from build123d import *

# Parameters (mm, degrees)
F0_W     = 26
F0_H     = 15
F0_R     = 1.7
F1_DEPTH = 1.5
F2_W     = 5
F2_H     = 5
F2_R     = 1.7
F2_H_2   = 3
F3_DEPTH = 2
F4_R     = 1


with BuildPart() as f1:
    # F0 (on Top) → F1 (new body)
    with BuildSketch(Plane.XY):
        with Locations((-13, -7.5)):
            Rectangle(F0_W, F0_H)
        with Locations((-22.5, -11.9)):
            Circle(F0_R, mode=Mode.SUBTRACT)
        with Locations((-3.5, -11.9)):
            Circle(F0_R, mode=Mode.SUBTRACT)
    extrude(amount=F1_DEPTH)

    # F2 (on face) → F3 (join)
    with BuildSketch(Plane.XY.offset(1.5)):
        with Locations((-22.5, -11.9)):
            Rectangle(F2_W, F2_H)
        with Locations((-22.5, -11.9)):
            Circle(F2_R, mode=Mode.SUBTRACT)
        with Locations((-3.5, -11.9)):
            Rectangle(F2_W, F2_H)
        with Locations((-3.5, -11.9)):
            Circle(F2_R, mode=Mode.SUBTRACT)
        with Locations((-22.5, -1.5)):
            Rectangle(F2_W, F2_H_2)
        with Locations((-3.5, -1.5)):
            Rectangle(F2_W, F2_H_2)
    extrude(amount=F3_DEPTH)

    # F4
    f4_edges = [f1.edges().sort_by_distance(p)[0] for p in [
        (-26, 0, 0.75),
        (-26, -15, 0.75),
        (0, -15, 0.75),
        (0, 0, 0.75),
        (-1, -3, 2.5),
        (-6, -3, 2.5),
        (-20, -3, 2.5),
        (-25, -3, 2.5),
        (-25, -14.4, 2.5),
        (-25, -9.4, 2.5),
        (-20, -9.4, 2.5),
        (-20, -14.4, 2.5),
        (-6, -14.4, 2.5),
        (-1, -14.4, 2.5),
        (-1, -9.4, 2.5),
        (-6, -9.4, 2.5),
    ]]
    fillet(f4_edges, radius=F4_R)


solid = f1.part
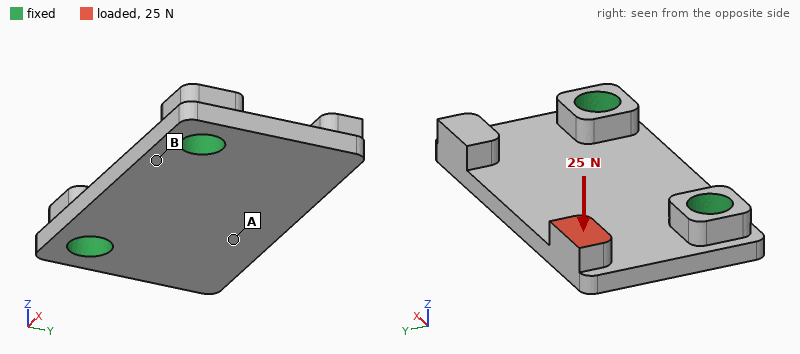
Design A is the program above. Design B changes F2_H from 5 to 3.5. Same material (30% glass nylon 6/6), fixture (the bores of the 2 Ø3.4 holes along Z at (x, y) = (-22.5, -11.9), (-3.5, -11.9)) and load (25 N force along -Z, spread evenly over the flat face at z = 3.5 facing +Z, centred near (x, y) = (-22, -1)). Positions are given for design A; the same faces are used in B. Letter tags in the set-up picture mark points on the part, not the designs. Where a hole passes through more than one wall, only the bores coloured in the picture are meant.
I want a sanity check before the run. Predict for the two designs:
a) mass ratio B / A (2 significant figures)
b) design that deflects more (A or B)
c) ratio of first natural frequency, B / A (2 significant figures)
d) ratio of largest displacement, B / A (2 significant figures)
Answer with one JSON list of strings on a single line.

["0.96", "B", "0.93", "1.1"]
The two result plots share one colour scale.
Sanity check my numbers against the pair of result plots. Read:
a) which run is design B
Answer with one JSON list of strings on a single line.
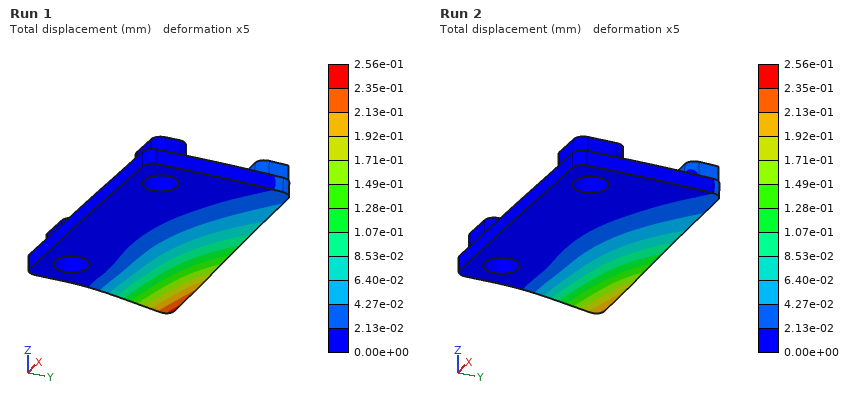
["Run 1"]
